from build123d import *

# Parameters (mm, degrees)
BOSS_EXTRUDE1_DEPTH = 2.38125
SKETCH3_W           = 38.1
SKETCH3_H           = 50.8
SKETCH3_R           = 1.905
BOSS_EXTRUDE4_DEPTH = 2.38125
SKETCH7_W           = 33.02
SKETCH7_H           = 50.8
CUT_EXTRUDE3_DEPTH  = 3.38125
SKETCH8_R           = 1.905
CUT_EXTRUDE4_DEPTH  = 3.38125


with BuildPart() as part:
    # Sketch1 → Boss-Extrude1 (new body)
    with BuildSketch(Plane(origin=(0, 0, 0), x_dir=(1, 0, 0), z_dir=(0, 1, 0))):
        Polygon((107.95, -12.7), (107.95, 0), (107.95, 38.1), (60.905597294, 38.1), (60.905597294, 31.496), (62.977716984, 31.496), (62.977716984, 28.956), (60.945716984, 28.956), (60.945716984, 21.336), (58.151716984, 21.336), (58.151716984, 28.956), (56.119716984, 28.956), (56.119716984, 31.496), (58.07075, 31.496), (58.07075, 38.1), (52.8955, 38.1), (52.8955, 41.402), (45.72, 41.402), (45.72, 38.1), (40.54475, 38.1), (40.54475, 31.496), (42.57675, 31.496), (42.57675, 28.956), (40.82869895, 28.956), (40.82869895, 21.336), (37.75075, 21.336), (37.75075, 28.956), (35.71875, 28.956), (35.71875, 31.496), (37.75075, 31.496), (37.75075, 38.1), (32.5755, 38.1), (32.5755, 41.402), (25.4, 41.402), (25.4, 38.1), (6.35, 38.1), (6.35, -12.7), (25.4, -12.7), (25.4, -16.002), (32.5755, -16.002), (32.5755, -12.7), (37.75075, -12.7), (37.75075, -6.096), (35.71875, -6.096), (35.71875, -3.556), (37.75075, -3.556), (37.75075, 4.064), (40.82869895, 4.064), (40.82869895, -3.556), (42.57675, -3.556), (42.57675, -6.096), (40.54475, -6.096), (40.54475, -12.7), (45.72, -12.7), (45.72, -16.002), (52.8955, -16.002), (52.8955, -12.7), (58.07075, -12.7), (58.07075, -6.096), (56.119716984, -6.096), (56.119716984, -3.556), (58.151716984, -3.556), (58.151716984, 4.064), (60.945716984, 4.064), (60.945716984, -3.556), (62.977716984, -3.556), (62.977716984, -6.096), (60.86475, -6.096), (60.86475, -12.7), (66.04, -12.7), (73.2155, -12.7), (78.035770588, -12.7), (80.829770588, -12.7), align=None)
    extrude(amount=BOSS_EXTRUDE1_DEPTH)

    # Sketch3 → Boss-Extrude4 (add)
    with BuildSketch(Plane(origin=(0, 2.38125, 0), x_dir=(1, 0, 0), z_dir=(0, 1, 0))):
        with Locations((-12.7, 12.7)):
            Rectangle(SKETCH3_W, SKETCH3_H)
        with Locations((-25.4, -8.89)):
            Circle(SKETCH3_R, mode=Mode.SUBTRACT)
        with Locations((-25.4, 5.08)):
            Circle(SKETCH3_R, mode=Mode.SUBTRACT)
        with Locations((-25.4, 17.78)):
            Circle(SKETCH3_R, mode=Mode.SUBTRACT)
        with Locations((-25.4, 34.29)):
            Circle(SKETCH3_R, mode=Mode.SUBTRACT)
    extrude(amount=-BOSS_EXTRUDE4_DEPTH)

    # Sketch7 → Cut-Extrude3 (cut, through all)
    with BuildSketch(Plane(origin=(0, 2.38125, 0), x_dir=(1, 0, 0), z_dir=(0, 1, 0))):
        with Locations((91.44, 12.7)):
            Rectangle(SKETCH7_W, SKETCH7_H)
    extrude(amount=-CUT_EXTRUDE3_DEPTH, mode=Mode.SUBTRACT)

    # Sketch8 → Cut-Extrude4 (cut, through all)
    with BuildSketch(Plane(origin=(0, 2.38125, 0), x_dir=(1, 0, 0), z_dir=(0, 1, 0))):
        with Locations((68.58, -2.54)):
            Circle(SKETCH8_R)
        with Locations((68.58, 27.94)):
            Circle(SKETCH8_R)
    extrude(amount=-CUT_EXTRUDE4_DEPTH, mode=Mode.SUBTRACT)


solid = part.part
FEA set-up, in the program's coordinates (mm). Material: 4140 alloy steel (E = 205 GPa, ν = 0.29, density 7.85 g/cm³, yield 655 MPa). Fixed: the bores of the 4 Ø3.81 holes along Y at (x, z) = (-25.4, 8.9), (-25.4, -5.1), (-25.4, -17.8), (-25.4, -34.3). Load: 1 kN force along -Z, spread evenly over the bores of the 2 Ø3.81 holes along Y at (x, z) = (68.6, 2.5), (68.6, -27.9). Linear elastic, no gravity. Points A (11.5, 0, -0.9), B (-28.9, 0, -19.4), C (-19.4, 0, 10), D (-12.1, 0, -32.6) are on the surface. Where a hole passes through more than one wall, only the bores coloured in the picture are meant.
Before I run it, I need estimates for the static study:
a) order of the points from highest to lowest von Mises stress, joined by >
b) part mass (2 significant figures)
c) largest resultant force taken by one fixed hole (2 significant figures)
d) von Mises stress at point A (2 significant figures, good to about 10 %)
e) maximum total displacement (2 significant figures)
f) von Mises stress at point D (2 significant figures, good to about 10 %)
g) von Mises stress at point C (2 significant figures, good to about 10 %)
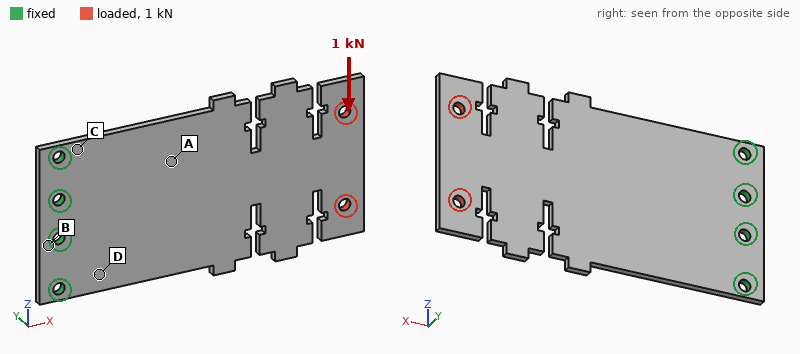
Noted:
C > D > A > B
97 g
2.0 kN
37 MPa
0.17 mm
64 MPa
90 MPa
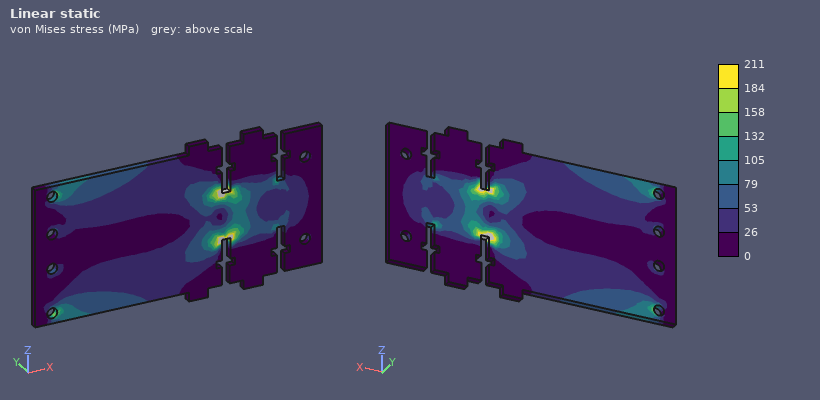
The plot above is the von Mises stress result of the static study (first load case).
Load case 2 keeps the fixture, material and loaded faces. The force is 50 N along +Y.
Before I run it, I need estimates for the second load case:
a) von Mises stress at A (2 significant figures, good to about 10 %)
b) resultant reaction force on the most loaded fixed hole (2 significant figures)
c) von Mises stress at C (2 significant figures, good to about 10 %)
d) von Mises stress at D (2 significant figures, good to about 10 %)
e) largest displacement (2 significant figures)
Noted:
58 MPa
42 N
86 MPa
81 MPa
1.4 mm
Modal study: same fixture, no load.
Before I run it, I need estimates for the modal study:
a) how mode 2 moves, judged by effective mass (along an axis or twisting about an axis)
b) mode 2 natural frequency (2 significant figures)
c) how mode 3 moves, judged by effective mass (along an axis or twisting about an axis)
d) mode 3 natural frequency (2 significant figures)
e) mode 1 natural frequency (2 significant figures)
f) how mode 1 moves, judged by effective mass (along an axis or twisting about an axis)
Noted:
twisting about X
740 Hz
along Y
1000 Hz
200 Hz
along Y
